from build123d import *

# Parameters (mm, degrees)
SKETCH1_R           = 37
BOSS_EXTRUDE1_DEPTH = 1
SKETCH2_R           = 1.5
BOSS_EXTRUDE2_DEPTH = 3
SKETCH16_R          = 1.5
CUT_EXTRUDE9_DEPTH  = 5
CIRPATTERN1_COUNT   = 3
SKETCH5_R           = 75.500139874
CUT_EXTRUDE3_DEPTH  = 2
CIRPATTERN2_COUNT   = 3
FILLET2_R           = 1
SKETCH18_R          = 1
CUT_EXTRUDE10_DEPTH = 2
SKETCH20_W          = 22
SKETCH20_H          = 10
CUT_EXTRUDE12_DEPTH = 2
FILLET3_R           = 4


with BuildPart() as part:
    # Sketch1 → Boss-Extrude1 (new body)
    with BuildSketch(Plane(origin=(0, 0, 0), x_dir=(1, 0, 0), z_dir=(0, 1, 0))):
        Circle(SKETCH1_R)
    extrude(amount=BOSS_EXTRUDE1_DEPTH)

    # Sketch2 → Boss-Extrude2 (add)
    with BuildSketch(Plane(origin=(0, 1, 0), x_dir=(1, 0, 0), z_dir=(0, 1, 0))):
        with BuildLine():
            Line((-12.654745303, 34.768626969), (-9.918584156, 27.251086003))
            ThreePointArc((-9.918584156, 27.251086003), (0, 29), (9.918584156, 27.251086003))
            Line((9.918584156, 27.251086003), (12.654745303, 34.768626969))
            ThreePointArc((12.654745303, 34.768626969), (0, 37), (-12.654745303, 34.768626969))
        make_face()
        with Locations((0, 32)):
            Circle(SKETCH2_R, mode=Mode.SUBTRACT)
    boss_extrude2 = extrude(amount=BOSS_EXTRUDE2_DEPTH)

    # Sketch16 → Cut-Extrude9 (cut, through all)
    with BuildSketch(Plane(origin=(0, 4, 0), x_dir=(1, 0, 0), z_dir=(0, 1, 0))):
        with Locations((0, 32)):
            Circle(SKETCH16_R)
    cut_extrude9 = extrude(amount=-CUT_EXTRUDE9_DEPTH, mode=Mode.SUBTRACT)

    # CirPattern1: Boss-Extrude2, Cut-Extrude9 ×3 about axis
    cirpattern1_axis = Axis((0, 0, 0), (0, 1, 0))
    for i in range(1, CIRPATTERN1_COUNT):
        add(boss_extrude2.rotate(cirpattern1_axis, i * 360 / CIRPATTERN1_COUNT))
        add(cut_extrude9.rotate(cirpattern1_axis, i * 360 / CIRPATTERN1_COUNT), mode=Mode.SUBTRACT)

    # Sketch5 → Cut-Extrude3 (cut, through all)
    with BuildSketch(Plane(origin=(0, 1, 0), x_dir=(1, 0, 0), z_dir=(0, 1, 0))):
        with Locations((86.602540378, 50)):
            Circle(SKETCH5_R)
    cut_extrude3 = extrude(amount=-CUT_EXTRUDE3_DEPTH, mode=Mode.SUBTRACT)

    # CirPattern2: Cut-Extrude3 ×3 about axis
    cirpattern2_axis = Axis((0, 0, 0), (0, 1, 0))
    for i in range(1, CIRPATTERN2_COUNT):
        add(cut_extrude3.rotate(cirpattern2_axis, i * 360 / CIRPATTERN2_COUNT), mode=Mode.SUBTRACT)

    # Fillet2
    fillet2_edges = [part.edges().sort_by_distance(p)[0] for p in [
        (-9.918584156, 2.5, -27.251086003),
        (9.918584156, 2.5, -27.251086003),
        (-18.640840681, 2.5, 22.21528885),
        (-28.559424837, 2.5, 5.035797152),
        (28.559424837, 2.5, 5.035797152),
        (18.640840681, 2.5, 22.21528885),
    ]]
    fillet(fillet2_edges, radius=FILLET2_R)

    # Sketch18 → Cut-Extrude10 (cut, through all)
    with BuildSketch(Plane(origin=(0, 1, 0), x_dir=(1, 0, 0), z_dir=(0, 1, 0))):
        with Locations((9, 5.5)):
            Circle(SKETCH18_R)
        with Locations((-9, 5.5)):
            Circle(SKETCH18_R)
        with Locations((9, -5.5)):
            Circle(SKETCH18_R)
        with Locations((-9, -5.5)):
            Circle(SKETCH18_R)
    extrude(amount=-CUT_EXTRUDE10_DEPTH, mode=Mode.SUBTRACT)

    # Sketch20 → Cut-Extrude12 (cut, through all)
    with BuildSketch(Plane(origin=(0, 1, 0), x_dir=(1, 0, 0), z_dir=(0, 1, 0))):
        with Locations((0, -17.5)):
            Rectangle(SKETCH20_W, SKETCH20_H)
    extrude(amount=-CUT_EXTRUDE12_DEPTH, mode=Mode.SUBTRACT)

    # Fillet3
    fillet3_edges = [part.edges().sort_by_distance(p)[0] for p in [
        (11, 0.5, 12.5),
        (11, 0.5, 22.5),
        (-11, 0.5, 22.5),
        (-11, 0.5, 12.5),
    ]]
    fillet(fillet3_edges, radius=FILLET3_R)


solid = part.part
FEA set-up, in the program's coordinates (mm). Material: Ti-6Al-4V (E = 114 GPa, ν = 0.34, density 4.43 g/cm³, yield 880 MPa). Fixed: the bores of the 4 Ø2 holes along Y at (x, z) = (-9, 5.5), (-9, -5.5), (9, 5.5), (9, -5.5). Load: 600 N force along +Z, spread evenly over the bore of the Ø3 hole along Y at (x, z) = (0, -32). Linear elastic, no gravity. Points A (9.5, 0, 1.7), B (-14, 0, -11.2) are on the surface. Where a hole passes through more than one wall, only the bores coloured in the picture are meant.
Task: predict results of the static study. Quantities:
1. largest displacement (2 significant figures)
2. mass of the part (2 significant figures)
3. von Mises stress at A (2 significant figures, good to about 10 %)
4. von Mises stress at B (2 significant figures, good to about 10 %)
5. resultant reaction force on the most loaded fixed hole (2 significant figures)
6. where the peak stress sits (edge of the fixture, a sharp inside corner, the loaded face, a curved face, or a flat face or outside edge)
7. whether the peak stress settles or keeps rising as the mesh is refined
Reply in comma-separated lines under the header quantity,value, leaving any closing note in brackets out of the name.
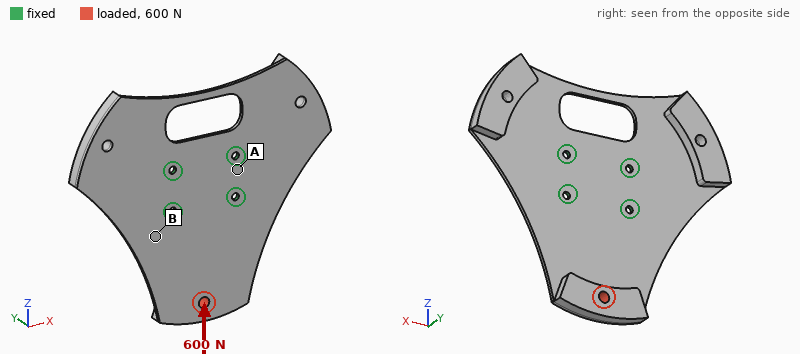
quantity,value
largest displacement,1.1 mm
mass of the part,20 g
von Mises stress at A,21 MPa
von Mises stress at B,110 MPa
resultant reaction force on the most loaded fixed hole,220 N
where the peak stress sits,edge of the fixture
whether the peak stress settles or keeps rising as the mesh is refined,keeps rising
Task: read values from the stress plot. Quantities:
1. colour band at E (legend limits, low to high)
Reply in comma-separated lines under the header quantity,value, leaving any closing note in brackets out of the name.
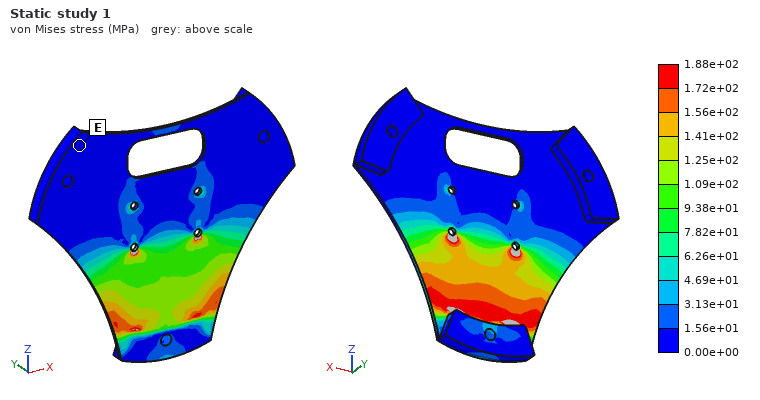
quantity,value
colour band at E,0.00e+00 to 1.56e+01 MPa
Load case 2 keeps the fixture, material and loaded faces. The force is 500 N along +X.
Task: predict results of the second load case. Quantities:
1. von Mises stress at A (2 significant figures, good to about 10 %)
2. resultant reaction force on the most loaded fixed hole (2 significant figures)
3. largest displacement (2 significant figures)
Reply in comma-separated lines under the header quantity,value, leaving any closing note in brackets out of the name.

quantity,value
von Mises stress at A,16 MPa
resultant reaction force on the most loaded fixed hole,530 N
largest displacement,0.21 mm
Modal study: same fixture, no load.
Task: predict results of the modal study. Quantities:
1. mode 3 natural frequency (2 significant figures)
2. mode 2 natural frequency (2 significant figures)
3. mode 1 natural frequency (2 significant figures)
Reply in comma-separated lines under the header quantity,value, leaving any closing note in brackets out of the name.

quantity,value
mode 3 natural frequency,690 Hz
mode 2 natural frequency,680 Hz
mode 1 natural frequency,620 Hz
